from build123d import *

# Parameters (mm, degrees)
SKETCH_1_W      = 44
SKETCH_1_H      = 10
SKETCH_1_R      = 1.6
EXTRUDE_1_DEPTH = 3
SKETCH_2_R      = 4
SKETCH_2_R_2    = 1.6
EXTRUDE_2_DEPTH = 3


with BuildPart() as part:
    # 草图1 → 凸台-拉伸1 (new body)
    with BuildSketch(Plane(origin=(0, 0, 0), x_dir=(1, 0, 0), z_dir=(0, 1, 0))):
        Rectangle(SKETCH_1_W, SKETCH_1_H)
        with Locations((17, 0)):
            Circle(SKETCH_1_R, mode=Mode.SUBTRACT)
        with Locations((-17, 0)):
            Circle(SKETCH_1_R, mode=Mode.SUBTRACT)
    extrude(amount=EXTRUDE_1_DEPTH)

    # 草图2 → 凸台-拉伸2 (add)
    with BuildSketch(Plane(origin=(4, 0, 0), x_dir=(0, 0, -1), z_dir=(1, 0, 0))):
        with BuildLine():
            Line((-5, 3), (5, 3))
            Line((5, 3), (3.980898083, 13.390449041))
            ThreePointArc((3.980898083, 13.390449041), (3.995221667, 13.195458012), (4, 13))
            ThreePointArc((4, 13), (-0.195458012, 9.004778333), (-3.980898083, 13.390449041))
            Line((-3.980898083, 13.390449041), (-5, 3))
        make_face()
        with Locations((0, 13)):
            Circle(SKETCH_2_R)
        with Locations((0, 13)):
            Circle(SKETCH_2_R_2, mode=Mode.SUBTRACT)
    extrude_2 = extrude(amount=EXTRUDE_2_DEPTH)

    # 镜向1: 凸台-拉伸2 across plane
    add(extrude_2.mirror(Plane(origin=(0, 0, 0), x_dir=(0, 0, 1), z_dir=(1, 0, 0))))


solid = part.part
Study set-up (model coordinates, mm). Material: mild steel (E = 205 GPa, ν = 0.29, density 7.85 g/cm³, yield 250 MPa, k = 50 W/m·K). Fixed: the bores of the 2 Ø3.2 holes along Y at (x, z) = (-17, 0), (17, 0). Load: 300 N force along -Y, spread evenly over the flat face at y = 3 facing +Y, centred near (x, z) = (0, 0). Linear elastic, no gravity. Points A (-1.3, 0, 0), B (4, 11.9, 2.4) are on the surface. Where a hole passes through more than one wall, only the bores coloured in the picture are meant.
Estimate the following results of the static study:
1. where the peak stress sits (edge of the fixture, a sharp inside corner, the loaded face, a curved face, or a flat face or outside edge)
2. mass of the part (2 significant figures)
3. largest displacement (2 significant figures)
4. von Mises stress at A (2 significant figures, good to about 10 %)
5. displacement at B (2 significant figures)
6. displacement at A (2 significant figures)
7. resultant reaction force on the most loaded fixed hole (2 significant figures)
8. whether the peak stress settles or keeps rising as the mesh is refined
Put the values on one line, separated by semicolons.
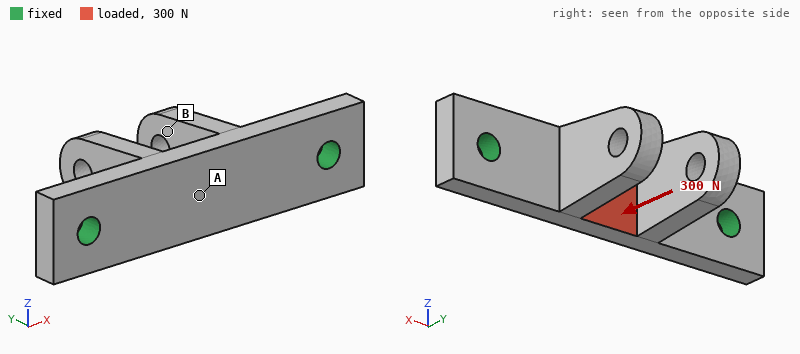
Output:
edge of the fixture; 15 g; 17 µm; 57 MPa; 14 µm; 11 µm; 150 N; keeps rising
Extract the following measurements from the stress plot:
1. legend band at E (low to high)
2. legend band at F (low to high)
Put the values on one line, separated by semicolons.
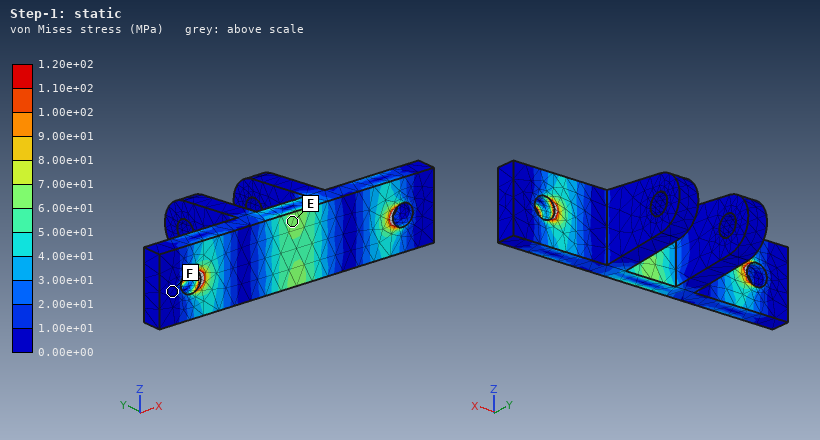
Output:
6.00e+01 to 7.00e+01 MPa; 0.00e+00 to 1.00e+01 MPa
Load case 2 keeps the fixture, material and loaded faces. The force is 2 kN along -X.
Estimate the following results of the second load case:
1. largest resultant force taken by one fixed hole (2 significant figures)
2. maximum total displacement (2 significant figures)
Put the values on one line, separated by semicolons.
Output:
1.0 kN; 4.1 µm
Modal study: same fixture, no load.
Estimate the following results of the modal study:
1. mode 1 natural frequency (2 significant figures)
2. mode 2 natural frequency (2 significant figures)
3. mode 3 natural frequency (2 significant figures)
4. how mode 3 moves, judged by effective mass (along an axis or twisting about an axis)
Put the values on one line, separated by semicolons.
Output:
8200 Hz; 8400 Hz; 12 kHz; along X
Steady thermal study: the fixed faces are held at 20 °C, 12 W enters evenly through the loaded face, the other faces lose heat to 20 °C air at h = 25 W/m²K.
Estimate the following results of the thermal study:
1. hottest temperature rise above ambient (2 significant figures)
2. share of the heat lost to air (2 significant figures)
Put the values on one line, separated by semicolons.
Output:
55 K; 9.6 %
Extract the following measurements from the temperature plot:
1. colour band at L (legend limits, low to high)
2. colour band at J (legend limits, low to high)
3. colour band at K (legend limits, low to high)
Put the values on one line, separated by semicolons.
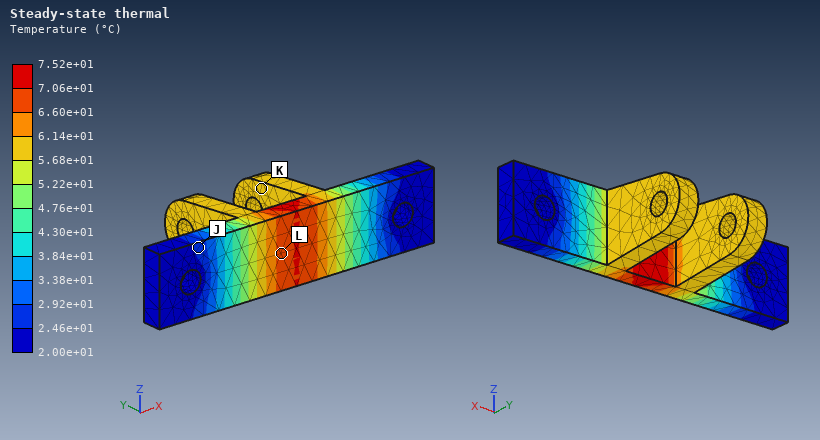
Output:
6.60e+01 to 7.06e+01 °C; 2.46e+01 to 2.92e+01 °C; 5.68e+01 to 6.14e+01 °C
